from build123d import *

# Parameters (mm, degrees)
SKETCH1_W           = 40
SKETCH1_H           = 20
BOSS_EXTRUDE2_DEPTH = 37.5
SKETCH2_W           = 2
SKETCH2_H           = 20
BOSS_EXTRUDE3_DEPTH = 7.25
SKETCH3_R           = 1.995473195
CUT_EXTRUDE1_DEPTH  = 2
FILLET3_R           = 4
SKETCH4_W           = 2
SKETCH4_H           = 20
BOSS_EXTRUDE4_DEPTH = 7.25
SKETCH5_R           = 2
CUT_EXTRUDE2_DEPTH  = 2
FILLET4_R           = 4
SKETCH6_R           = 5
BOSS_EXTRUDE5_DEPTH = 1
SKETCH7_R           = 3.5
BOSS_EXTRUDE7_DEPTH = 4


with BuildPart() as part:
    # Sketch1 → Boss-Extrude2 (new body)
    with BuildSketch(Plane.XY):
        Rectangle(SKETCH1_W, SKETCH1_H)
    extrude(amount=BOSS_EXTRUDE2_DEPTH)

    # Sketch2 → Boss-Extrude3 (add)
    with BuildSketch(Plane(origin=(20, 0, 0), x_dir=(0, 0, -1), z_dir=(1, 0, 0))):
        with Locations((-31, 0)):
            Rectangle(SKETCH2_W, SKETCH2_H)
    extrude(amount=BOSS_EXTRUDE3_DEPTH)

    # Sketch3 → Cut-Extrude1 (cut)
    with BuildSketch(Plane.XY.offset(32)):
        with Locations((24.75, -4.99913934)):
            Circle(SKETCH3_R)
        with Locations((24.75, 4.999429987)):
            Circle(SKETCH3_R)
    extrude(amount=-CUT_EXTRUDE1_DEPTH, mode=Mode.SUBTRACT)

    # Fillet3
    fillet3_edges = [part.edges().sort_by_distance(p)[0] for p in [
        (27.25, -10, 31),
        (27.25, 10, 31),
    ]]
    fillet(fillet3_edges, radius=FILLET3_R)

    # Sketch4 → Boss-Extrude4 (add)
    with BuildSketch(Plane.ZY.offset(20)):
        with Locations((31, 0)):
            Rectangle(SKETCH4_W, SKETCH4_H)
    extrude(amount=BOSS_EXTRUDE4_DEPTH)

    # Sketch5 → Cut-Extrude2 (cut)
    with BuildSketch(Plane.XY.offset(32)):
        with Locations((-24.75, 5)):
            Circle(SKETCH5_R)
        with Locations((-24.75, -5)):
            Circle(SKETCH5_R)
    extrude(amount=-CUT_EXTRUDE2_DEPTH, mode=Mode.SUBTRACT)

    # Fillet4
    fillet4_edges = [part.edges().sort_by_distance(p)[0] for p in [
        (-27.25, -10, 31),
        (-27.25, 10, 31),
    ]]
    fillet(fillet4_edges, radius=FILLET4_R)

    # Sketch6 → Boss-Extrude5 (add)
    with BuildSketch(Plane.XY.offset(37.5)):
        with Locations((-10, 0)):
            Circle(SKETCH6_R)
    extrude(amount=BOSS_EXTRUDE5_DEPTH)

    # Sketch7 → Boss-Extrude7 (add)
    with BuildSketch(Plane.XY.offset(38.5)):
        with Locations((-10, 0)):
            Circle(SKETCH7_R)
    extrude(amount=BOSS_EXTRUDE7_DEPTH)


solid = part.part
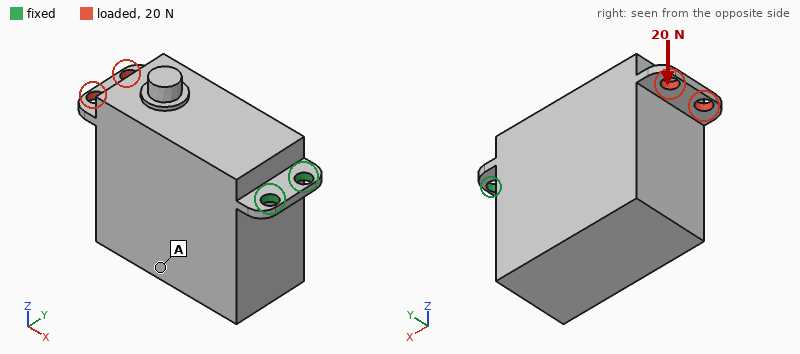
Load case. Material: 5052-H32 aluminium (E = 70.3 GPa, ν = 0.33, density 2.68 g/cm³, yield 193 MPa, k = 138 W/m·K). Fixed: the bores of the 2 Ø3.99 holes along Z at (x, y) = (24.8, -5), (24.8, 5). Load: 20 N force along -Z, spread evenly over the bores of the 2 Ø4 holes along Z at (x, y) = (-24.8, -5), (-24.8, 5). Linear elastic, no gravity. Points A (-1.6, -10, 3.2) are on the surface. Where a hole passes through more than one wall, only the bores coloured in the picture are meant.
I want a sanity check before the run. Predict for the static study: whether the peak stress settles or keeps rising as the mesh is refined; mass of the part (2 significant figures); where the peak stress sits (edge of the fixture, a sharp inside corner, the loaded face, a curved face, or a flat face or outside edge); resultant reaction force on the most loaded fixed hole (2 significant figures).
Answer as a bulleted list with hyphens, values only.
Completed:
- keeps rising
- 82 g
- edge of the fixture
- 10 N
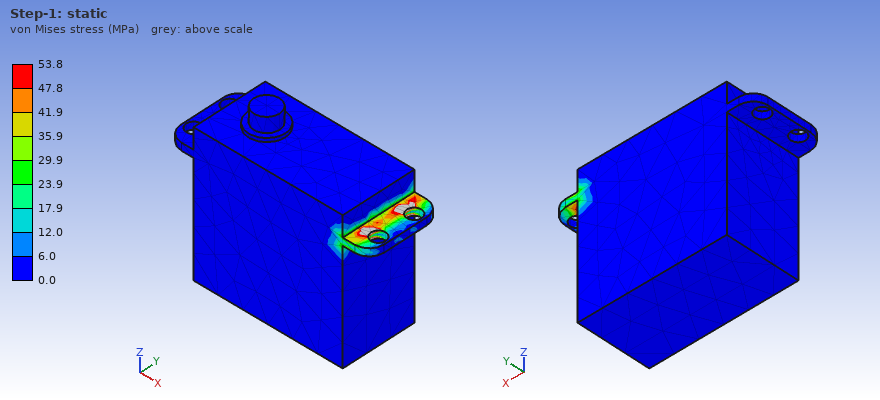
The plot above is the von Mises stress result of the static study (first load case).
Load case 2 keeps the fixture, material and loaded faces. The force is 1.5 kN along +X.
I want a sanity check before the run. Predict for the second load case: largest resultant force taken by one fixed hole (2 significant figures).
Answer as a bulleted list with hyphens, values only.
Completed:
- 750 N
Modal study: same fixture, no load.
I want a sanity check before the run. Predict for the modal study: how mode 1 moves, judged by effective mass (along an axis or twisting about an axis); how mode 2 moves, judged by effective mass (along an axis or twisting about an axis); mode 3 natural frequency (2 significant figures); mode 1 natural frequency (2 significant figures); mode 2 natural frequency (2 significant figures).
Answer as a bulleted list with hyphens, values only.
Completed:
- along Z
- along Y
- 3100 Hz
- 300 Hz
- 1500 Hz
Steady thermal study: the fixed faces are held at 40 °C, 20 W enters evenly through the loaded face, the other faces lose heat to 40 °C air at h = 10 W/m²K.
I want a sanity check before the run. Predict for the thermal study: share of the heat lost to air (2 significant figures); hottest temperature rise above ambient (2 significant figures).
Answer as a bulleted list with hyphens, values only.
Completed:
- 7.8 %
- 65 K
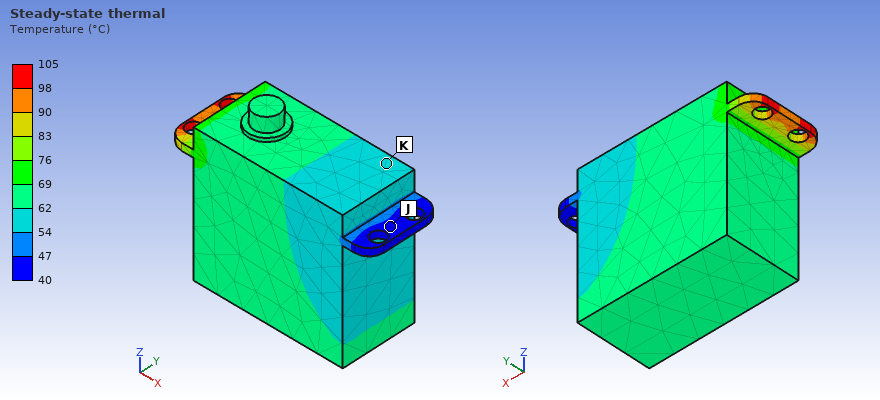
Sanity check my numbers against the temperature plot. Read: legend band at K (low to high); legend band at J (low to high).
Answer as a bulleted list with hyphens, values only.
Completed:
- 54 to 62 °C
- 40 to 47 °C
